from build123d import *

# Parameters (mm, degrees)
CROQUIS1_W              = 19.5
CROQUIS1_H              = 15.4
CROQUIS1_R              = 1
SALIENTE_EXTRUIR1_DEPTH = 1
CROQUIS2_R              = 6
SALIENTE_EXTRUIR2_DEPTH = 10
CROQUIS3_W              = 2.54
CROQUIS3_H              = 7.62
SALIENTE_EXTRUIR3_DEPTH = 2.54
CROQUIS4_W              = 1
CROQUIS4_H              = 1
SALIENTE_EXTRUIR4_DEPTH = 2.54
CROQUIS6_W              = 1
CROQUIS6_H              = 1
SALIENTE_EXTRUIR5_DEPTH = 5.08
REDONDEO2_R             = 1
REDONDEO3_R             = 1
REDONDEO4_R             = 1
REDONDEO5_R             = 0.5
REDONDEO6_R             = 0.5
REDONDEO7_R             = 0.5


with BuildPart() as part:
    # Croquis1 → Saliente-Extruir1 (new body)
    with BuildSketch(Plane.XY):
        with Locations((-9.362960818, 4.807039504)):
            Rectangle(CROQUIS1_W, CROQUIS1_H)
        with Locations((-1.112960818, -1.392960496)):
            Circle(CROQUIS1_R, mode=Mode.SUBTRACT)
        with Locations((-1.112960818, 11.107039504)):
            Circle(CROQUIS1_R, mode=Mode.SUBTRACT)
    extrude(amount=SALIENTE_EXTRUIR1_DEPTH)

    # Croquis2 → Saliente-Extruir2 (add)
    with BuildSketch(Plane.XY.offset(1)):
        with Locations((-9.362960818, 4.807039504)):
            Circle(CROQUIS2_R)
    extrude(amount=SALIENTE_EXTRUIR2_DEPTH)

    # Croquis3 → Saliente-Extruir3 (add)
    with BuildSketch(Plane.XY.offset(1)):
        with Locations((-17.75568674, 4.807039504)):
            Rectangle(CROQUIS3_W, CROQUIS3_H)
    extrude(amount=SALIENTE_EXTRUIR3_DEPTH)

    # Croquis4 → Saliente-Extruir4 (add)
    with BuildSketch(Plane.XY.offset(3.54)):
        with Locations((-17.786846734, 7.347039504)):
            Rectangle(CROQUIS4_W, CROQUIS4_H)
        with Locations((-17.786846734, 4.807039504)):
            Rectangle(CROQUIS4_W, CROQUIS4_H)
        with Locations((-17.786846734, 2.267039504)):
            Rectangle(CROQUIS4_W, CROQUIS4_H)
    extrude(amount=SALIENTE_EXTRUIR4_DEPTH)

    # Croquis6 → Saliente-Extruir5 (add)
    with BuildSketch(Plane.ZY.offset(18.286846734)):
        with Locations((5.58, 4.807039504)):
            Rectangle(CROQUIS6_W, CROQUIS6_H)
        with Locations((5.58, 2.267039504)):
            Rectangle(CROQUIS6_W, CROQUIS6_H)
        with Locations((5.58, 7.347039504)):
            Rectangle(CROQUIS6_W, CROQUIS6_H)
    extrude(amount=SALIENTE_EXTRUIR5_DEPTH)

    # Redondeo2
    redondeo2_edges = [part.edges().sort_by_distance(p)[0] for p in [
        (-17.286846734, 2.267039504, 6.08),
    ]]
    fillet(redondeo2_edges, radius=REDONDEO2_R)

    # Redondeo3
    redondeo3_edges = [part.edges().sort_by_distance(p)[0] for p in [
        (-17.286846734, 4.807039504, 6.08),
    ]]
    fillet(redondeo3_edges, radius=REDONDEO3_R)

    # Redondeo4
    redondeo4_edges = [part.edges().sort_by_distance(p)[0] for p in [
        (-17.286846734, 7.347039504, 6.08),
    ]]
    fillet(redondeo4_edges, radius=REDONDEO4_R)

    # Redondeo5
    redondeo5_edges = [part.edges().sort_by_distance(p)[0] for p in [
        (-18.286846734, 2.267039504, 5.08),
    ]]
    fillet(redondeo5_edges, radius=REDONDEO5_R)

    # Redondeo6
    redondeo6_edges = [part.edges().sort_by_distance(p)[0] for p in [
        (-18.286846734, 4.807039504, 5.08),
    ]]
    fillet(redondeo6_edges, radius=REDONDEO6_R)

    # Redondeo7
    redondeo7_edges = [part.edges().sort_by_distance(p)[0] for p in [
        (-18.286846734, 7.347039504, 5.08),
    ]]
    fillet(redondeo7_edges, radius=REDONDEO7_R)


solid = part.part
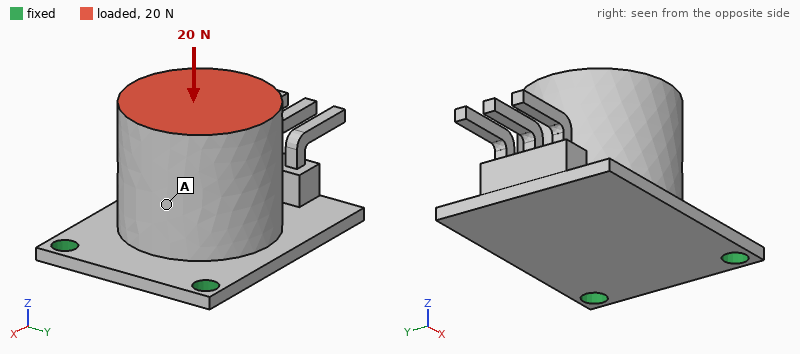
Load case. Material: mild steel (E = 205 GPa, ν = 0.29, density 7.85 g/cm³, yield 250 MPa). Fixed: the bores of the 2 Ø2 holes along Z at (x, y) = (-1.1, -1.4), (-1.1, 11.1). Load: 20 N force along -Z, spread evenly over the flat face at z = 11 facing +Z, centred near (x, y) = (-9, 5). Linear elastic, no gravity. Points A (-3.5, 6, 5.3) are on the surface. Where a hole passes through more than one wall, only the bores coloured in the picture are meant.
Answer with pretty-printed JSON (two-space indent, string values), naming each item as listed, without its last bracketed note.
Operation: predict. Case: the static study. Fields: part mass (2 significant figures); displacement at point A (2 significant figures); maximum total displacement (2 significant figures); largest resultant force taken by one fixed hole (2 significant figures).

{
  "part mass": "12 g",
  "displacement at point A": "7.8 µm",
  "maximum total displacement": "35 µm",
  "largest resultant force taken by one fixed hole": "10 N"
}
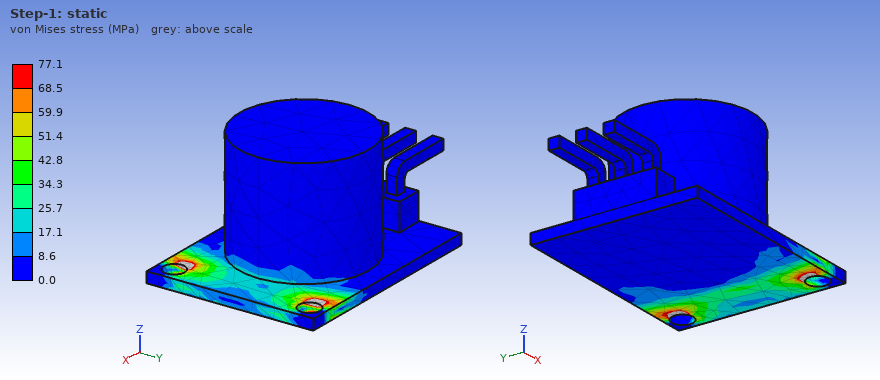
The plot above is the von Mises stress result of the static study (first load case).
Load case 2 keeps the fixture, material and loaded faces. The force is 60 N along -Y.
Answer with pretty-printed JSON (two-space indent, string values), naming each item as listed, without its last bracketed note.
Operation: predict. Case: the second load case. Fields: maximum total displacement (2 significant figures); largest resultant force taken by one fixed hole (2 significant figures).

{
  "maximum total displacement": "12 µm",
  "largest resultant force taken by one fixed hole": "76 N"
}
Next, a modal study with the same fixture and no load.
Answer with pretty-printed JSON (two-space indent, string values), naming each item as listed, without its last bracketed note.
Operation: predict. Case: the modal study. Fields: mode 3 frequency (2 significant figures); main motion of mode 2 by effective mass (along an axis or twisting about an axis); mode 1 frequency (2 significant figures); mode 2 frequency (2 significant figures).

{
  "mode 3 frequency": "11 kHz",
  "main motion of mode 2 by effective mass": "along Y",
  "mode 1 frequency": "1300 Hz",
  "mode 2 frequency": "5800 Hz"
}
